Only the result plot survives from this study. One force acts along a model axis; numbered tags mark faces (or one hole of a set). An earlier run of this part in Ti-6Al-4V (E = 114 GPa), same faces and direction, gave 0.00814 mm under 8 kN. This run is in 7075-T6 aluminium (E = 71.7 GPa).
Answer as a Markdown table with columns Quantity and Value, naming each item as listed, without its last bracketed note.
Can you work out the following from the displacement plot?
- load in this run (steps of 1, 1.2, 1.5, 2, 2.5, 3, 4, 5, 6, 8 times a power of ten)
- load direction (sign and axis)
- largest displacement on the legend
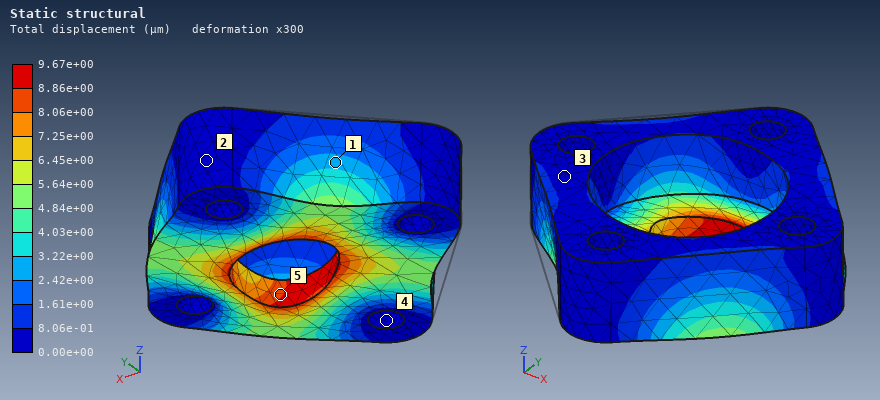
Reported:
| Quantity | Value |
|---|---|
| load in this run | 6 kN |
| load direction | +X |
| largest displacement on the legend | 9.67e+00 µm |
